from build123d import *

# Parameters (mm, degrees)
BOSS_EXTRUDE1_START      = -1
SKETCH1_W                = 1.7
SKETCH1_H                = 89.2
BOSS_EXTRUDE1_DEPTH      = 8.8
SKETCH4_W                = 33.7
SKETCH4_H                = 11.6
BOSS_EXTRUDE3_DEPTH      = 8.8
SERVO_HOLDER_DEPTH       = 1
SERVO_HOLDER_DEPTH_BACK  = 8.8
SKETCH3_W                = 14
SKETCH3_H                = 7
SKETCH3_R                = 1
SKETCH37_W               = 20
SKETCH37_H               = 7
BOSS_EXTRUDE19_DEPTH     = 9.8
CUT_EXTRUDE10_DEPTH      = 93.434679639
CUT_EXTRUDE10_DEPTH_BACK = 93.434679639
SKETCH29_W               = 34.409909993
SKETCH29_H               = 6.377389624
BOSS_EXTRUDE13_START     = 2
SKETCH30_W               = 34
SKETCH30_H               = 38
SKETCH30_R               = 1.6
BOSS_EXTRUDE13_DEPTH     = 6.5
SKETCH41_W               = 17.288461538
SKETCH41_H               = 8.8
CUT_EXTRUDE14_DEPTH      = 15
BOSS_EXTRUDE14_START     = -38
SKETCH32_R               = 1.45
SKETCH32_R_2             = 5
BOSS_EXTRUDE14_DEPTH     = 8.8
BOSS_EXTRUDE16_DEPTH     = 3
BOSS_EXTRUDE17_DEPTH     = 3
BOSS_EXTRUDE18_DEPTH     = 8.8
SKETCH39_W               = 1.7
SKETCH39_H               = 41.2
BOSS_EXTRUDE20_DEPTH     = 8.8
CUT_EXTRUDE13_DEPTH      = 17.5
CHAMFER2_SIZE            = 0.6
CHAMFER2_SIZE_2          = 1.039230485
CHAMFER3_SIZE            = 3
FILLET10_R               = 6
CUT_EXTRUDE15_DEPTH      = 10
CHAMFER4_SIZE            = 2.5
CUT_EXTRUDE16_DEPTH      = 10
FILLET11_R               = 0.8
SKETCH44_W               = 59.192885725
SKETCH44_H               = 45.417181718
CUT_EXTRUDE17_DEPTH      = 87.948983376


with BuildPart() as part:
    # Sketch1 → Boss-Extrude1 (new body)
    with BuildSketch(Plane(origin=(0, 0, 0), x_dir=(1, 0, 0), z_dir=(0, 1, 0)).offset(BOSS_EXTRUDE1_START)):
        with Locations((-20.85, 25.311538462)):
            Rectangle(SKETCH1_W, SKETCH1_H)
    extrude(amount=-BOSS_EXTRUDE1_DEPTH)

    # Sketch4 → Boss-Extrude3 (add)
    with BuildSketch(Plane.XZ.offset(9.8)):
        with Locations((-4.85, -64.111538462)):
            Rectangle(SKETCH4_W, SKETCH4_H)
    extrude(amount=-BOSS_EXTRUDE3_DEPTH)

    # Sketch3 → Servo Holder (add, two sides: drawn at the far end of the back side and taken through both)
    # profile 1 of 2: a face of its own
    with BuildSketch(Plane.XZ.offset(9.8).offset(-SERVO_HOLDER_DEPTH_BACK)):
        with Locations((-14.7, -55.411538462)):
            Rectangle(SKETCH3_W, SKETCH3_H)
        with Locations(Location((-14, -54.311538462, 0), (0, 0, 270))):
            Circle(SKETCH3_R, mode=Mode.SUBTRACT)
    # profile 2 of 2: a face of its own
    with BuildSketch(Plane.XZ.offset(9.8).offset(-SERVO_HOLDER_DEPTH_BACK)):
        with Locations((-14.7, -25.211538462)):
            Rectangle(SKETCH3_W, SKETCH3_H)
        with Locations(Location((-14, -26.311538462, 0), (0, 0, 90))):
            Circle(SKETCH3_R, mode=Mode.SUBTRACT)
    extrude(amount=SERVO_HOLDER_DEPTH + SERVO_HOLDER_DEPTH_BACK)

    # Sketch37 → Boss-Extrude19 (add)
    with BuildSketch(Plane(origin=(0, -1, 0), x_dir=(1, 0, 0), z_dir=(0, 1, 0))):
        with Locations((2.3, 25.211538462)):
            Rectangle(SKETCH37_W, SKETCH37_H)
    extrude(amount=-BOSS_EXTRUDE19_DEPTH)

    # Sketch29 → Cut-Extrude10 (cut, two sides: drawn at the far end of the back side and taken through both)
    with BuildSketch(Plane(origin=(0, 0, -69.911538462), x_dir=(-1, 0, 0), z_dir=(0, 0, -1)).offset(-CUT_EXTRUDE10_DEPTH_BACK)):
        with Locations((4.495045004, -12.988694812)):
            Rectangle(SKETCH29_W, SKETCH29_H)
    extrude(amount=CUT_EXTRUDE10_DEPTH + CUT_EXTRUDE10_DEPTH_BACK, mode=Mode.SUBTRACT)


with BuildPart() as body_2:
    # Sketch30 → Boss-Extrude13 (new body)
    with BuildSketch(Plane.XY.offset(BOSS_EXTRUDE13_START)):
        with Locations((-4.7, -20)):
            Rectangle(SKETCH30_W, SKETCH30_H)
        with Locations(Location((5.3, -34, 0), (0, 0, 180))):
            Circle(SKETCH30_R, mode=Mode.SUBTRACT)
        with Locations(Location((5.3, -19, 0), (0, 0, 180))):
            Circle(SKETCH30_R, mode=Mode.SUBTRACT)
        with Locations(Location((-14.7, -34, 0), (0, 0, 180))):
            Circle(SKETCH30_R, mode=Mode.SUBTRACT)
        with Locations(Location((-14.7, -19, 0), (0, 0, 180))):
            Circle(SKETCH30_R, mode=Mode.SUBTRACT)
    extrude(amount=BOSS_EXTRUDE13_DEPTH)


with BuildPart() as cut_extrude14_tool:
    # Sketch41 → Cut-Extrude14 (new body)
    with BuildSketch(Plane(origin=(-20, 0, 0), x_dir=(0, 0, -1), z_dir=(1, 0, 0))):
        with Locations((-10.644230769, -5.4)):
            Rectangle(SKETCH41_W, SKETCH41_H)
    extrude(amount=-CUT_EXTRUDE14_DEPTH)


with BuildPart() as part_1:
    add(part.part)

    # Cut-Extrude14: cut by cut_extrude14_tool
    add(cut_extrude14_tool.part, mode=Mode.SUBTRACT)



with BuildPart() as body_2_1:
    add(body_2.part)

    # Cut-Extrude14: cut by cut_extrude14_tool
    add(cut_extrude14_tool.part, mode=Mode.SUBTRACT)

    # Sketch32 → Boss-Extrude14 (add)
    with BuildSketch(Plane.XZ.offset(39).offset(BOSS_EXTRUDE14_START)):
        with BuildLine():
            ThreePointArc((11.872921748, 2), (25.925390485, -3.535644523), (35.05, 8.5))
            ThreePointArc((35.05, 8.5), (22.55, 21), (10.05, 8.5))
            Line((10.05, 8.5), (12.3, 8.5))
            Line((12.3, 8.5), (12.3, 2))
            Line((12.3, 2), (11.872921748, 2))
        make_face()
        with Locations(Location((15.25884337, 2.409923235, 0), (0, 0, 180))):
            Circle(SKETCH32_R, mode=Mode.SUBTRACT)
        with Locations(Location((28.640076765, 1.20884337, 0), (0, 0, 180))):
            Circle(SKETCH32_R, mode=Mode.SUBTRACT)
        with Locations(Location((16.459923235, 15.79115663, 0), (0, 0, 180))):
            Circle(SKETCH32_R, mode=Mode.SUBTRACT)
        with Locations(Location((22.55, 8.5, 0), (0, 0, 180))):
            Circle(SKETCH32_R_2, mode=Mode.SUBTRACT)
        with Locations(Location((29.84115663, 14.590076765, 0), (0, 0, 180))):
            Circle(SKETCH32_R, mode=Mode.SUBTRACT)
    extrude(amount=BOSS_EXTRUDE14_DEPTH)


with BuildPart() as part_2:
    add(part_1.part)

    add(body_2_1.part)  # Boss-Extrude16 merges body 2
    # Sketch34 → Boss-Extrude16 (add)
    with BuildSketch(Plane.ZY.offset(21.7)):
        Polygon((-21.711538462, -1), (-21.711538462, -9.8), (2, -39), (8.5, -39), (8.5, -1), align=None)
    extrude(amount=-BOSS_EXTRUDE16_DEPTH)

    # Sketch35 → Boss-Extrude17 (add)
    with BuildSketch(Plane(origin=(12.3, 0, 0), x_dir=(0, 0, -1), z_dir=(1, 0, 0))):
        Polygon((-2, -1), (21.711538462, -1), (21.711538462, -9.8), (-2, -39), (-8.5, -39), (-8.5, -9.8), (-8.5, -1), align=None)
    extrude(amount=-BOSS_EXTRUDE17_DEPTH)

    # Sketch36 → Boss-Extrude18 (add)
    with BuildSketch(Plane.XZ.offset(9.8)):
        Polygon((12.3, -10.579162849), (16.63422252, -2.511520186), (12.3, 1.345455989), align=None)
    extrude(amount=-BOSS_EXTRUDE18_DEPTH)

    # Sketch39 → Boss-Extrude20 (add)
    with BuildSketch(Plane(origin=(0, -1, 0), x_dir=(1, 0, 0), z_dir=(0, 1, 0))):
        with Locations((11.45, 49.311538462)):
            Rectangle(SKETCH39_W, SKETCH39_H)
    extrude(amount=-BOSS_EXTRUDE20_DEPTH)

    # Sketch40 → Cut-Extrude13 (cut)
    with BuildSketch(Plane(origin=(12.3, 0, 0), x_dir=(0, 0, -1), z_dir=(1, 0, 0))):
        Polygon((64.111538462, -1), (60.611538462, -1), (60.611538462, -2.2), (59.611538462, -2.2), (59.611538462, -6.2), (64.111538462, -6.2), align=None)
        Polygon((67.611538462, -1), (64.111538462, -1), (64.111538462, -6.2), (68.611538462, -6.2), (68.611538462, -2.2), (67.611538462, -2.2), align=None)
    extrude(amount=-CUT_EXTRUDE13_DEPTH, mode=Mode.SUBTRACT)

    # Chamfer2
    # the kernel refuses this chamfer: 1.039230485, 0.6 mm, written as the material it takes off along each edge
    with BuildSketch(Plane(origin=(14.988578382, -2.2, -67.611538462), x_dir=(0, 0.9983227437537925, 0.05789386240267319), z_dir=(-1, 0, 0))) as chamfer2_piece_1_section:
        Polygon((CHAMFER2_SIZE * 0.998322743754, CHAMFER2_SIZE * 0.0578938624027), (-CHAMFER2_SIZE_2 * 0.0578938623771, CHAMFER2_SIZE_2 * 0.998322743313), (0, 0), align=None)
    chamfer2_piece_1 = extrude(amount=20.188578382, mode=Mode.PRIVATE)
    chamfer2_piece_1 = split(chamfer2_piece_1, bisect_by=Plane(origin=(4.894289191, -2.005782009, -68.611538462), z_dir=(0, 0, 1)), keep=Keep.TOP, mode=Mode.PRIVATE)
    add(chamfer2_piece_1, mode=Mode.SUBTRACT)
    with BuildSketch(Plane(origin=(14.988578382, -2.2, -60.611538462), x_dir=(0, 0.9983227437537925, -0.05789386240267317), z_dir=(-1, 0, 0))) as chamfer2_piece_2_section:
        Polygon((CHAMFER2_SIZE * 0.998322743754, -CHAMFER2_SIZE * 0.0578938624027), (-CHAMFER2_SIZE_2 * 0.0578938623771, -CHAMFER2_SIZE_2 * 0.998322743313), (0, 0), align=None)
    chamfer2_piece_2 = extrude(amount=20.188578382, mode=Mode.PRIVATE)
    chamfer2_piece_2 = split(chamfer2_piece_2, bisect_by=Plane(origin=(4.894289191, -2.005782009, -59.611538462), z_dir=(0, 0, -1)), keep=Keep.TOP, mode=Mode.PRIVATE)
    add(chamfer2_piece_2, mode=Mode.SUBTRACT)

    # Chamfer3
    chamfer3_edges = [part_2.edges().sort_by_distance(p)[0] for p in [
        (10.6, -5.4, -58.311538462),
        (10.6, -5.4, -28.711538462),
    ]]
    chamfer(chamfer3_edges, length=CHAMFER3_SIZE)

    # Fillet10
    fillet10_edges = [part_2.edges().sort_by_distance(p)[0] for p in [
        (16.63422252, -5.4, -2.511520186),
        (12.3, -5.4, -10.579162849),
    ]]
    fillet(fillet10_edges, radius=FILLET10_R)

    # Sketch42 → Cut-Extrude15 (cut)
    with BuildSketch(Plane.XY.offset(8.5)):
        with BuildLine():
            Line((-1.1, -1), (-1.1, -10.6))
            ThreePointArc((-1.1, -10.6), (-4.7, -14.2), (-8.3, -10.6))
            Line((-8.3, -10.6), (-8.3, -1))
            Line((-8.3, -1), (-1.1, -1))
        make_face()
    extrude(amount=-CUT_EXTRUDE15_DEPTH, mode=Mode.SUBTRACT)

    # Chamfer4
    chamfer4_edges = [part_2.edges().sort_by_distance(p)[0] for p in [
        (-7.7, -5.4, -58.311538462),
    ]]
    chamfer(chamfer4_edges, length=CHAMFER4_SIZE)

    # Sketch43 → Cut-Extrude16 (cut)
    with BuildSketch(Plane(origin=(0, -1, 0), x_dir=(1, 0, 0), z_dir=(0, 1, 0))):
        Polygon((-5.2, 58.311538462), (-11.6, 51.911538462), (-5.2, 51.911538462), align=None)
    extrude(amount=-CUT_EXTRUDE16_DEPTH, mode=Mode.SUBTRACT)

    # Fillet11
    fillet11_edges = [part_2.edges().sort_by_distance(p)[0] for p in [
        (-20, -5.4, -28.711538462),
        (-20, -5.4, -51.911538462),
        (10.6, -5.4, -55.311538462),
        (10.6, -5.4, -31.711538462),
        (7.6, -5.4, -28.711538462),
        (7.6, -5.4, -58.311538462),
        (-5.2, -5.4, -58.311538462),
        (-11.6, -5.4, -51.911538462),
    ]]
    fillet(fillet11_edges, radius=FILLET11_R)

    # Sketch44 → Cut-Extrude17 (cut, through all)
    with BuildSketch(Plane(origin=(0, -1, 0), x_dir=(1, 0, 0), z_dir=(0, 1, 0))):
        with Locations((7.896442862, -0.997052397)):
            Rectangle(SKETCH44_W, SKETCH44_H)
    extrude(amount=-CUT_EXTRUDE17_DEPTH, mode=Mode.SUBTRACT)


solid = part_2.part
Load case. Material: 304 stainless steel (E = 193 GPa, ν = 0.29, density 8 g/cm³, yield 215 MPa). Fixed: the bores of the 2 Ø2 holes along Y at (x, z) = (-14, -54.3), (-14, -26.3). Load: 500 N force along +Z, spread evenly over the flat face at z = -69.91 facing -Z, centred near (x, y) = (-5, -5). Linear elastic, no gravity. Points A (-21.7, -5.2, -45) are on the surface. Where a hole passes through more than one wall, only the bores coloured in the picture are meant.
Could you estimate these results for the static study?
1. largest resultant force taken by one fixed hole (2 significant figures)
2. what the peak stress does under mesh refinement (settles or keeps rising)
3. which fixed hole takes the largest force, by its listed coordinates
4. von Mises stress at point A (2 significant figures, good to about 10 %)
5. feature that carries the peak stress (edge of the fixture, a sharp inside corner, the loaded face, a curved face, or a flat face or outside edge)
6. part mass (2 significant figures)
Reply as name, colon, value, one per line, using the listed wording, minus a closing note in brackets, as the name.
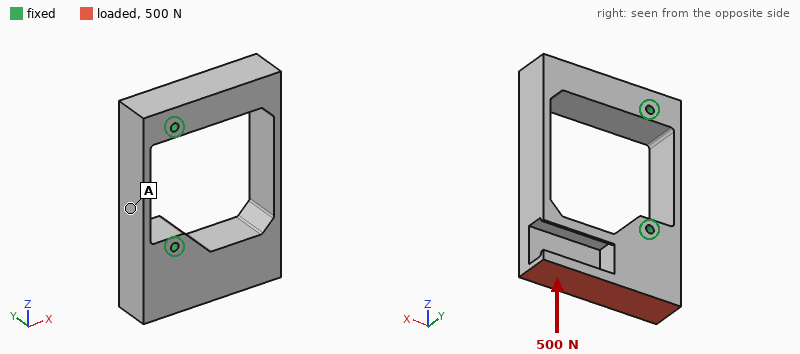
largest resultant force taken by one fixed hole: 500 N
what the peak stress does under mesh refinement: keeps rising
which fixed hole takes the largest force, by its listed coordinates: (-14, -54.3)
von Mises stress at point A: 8.9 MPa
feature that carries the peak stress: edge of the fixture
part mass: 51 g
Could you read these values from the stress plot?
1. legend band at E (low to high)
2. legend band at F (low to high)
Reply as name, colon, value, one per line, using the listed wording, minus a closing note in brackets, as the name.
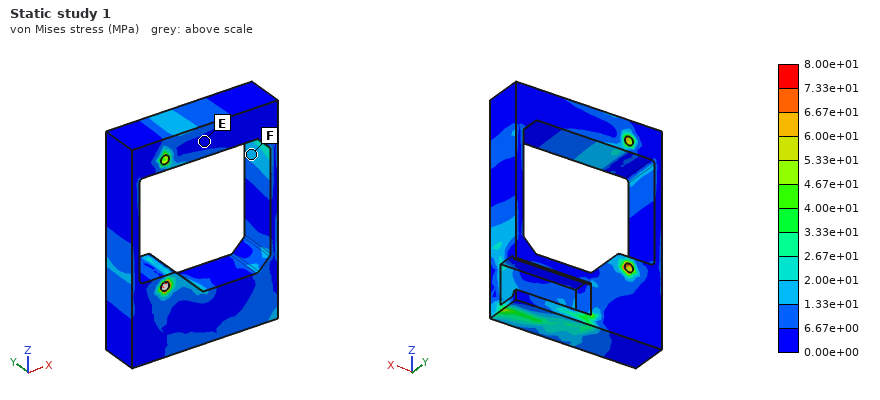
legend band at E: 0.00e+00 to 6.67e+00 MPa
legend band at F: 1.33e+01 to 2.00e+01 MPa
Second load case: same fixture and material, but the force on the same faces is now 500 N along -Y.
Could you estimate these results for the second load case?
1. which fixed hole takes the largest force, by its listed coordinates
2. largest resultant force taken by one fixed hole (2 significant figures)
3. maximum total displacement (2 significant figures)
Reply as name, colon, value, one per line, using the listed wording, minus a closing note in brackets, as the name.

which fixed hole takes the largest force, by its listed coordinates: (-14, -54.3)
largest resultant force taken by one fixed hole: 530 N
maximum total displacement: 28 µm
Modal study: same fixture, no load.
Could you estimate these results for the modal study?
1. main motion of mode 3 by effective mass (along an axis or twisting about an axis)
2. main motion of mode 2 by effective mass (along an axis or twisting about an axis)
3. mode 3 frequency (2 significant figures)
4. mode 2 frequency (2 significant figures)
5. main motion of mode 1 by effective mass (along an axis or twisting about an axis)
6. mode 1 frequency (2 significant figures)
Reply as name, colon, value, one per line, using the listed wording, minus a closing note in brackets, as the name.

main motion of mode 3 by effective mass: twisting about X
main motion of mode 2 by effective mass: along Y
mode 3 frequency: 8500 Hz
mode 2 frequency: 6800 Hz
main motion of mode 1 by effective mass: along Z
mode 1 frequency: 5100 Hz
